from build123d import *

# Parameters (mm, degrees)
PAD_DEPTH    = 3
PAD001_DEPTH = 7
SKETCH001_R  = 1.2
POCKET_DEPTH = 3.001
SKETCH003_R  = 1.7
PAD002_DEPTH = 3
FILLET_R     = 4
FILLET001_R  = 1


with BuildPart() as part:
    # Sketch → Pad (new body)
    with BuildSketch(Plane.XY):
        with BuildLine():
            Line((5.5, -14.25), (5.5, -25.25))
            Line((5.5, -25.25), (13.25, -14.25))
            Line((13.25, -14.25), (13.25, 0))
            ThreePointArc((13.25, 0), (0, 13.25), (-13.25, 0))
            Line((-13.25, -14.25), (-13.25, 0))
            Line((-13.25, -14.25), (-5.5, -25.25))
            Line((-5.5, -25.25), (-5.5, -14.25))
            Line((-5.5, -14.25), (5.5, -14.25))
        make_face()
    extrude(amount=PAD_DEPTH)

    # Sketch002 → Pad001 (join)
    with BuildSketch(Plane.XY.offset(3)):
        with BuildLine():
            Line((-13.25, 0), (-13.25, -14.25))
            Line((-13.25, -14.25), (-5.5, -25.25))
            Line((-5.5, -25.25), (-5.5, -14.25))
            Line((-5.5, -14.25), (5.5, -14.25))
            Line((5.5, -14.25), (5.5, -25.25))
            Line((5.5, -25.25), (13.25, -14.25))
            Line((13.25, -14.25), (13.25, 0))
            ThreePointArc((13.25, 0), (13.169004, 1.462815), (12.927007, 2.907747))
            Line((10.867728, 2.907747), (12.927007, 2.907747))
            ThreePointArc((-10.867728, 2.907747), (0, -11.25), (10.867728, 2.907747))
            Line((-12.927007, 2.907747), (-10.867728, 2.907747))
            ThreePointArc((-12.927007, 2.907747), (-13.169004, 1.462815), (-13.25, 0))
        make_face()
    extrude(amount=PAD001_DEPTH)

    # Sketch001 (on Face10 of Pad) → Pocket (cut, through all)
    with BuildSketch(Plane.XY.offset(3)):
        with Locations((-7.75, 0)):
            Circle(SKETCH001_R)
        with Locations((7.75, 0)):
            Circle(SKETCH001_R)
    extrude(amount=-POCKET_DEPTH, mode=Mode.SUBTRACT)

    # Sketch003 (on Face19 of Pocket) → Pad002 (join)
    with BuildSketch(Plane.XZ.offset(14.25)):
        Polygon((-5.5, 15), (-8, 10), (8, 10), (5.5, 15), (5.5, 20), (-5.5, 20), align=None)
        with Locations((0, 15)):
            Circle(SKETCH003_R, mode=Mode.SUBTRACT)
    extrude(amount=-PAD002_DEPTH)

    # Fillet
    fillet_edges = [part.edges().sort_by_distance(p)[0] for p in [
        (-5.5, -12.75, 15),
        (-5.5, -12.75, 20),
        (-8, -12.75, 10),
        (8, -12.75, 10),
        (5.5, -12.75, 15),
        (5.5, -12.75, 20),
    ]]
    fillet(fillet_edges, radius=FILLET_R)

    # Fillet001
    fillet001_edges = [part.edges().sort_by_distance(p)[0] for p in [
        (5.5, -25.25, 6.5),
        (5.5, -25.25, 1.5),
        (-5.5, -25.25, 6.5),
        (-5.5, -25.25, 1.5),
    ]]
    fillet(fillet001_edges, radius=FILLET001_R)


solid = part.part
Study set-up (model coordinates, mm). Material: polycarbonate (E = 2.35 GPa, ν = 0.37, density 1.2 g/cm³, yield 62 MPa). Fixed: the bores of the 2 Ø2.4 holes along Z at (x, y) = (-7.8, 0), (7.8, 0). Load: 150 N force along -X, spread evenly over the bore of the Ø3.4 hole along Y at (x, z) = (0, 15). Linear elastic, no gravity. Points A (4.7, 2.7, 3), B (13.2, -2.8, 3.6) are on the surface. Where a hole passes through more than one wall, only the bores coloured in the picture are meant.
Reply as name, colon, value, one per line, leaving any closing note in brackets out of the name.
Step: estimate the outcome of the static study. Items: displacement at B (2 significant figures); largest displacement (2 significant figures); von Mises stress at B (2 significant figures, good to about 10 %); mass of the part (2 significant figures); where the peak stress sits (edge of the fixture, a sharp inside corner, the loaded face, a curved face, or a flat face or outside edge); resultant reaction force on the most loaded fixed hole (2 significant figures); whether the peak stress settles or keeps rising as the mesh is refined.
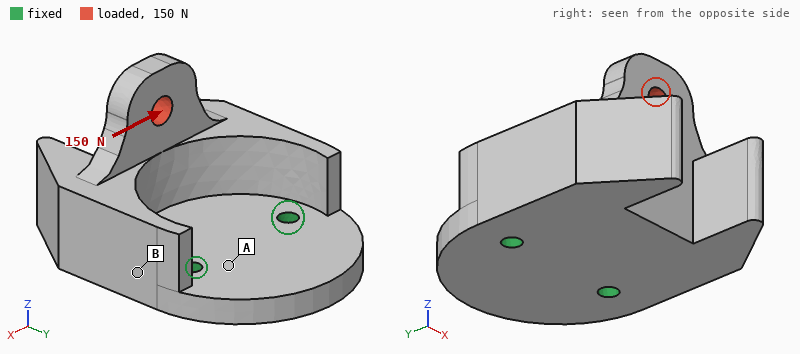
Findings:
displacement at B: 0.13 mm
largest displacement: 0.51 mm
von Mises stress at B: 8.9 MPa
mass of the part: 5.3 g
where the peak stress sits: edge of the fixture
resultant reaction force on the most loaded fixed hole: 170 N
whether the peak stress settles or keeps rising as the mesh is refined: keeps rising
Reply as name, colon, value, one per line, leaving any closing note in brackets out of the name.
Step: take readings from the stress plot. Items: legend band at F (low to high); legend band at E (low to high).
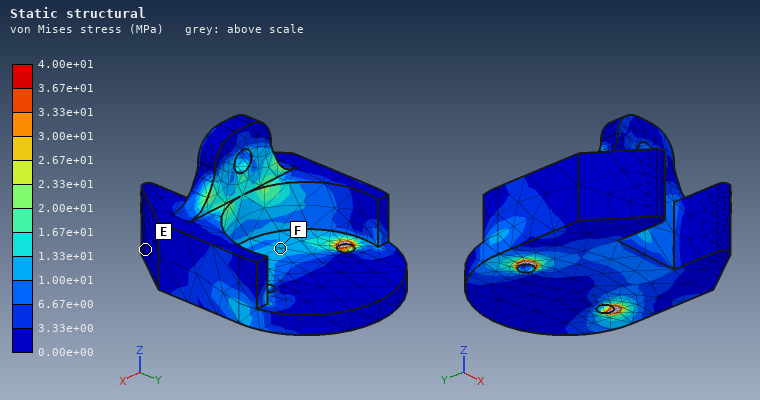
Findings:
legend band at F: 1.00e+01 to 1.33e+01 MPa
legend band at E: 0.00e+00 to 3.33e+00 MPa
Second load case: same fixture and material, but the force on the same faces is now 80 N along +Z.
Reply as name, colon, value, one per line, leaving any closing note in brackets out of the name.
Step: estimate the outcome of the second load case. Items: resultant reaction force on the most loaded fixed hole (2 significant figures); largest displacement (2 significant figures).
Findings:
resultant reaction force on the most loaded fixed hole: 41 N
largest displacement: 0.50 mm
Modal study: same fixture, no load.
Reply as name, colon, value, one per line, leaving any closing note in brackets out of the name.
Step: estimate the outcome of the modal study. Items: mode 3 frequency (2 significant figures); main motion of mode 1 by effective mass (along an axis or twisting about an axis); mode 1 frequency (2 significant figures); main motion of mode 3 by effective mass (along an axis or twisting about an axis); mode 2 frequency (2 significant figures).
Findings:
mode 3 frequency: 4500 Hz
main motion of mode 1 by effective mass: along Z
mode 1 frequency: 1300 Hz
main motion of mode 3 by effective mass: along X
mode 2 frequency: 2400 Hz
